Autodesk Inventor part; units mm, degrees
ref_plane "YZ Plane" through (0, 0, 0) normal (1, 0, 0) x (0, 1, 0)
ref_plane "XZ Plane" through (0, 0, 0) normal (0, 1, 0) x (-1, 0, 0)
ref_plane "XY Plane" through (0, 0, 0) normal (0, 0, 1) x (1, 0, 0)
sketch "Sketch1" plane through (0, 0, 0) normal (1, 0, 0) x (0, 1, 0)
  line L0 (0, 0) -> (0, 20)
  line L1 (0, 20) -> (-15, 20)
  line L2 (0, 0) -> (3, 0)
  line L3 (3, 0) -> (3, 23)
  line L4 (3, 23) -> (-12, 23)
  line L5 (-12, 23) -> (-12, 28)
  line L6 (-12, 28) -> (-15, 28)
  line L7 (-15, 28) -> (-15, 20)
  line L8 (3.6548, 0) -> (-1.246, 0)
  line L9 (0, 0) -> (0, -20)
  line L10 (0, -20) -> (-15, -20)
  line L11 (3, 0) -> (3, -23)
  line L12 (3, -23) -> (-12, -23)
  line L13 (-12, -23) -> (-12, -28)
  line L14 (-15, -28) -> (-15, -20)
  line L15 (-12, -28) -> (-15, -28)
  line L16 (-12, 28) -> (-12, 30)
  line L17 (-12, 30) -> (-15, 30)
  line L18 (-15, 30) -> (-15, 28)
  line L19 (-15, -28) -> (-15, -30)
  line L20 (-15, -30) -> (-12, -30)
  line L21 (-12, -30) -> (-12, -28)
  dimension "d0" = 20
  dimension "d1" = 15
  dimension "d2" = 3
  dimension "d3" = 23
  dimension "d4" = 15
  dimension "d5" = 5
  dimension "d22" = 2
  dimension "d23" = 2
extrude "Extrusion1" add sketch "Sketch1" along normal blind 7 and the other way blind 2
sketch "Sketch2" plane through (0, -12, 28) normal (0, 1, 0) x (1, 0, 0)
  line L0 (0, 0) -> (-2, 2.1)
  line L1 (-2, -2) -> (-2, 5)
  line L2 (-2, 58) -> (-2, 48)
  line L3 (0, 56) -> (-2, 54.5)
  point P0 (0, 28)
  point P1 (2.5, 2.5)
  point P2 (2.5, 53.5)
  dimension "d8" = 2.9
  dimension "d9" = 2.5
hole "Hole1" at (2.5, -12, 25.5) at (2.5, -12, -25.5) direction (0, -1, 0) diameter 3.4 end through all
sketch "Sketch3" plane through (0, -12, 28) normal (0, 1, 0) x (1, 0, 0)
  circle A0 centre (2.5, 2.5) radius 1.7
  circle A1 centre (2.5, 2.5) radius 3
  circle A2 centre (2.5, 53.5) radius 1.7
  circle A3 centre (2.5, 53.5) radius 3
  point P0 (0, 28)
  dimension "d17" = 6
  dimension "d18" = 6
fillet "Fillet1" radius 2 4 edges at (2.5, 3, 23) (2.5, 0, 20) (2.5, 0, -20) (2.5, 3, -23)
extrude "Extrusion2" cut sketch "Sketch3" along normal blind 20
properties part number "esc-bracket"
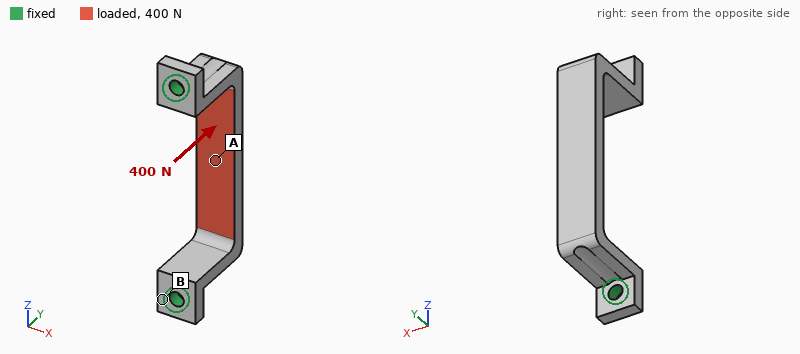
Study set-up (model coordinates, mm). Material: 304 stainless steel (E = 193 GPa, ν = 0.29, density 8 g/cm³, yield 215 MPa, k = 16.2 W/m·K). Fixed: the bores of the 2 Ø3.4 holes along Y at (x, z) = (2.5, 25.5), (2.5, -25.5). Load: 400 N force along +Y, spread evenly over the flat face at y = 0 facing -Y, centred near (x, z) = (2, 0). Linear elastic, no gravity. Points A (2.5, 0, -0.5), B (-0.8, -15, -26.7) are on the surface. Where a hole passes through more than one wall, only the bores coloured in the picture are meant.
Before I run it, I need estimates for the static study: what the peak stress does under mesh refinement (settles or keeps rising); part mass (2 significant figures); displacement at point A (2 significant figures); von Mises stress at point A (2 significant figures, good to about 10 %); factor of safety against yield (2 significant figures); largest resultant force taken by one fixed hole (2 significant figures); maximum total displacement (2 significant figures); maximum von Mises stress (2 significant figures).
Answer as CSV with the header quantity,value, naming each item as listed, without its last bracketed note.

quantity,value
what the peak stress does under mesh refinement,settles
part mass,19 g
displacement at point A,33 µm
von Mises stress at point A,64 MPa
factor of safety against yield,1.8
largest resultant force taken by one fixed hole,250 N
maximum total displacement,34 µm
maximum von Mises stress,120 MPa
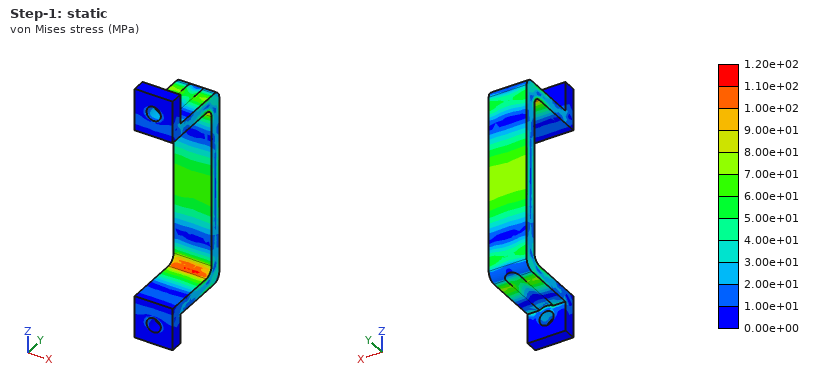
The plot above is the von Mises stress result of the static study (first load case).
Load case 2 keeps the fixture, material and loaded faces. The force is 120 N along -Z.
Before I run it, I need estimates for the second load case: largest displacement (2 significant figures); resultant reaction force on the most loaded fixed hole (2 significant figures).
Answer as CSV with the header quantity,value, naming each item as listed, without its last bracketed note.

quantity,value
largest displacement,11 µm
resultant reaction force on the most loaded fixed hole,62 N
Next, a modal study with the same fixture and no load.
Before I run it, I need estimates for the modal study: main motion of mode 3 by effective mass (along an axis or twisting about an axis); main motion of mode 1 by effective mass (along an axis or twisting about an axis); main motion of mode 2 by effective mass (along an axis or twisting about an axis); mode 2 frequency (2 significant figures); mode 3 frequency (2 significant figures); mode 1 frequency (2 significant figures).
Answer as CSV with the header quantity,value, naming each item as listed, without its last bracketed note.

quantity,value
main motion of mode 3 by effective mass,along Y
main motion of mode 1 by effective mass,along Z
main motion of mode 2 by effective mass,along X
mode 2 frequency,5400 Hz
mode 3 frequency,7000 Hz
mode 1 frequency,5000 Hz
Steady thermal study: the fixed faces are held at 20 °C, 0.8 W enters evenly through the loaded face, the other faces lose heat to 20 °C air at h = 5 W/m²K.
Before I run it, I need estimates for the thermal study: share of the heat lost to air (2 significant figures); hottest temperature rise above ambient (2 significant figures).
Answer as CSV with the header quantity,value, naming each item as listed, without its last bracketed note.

quantity,value
share of the heat lost to air,12 %
hottest temperature rise above ambient,23 K
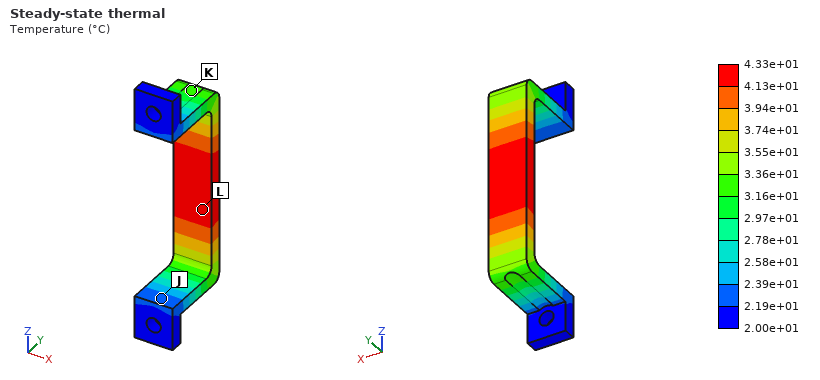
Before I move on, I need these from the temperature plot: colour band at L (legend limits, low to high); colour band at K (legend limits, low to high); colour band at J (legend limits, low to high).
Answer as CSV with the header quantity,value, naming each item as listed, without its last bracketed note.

quantity,value
colour band at L,4.13e+01 to 4.33e+01 °C
colour band at K,3.16e+01 to 3.36e+01 °C
colour band at J,2.19e+01 to 2.39e+01 °C
